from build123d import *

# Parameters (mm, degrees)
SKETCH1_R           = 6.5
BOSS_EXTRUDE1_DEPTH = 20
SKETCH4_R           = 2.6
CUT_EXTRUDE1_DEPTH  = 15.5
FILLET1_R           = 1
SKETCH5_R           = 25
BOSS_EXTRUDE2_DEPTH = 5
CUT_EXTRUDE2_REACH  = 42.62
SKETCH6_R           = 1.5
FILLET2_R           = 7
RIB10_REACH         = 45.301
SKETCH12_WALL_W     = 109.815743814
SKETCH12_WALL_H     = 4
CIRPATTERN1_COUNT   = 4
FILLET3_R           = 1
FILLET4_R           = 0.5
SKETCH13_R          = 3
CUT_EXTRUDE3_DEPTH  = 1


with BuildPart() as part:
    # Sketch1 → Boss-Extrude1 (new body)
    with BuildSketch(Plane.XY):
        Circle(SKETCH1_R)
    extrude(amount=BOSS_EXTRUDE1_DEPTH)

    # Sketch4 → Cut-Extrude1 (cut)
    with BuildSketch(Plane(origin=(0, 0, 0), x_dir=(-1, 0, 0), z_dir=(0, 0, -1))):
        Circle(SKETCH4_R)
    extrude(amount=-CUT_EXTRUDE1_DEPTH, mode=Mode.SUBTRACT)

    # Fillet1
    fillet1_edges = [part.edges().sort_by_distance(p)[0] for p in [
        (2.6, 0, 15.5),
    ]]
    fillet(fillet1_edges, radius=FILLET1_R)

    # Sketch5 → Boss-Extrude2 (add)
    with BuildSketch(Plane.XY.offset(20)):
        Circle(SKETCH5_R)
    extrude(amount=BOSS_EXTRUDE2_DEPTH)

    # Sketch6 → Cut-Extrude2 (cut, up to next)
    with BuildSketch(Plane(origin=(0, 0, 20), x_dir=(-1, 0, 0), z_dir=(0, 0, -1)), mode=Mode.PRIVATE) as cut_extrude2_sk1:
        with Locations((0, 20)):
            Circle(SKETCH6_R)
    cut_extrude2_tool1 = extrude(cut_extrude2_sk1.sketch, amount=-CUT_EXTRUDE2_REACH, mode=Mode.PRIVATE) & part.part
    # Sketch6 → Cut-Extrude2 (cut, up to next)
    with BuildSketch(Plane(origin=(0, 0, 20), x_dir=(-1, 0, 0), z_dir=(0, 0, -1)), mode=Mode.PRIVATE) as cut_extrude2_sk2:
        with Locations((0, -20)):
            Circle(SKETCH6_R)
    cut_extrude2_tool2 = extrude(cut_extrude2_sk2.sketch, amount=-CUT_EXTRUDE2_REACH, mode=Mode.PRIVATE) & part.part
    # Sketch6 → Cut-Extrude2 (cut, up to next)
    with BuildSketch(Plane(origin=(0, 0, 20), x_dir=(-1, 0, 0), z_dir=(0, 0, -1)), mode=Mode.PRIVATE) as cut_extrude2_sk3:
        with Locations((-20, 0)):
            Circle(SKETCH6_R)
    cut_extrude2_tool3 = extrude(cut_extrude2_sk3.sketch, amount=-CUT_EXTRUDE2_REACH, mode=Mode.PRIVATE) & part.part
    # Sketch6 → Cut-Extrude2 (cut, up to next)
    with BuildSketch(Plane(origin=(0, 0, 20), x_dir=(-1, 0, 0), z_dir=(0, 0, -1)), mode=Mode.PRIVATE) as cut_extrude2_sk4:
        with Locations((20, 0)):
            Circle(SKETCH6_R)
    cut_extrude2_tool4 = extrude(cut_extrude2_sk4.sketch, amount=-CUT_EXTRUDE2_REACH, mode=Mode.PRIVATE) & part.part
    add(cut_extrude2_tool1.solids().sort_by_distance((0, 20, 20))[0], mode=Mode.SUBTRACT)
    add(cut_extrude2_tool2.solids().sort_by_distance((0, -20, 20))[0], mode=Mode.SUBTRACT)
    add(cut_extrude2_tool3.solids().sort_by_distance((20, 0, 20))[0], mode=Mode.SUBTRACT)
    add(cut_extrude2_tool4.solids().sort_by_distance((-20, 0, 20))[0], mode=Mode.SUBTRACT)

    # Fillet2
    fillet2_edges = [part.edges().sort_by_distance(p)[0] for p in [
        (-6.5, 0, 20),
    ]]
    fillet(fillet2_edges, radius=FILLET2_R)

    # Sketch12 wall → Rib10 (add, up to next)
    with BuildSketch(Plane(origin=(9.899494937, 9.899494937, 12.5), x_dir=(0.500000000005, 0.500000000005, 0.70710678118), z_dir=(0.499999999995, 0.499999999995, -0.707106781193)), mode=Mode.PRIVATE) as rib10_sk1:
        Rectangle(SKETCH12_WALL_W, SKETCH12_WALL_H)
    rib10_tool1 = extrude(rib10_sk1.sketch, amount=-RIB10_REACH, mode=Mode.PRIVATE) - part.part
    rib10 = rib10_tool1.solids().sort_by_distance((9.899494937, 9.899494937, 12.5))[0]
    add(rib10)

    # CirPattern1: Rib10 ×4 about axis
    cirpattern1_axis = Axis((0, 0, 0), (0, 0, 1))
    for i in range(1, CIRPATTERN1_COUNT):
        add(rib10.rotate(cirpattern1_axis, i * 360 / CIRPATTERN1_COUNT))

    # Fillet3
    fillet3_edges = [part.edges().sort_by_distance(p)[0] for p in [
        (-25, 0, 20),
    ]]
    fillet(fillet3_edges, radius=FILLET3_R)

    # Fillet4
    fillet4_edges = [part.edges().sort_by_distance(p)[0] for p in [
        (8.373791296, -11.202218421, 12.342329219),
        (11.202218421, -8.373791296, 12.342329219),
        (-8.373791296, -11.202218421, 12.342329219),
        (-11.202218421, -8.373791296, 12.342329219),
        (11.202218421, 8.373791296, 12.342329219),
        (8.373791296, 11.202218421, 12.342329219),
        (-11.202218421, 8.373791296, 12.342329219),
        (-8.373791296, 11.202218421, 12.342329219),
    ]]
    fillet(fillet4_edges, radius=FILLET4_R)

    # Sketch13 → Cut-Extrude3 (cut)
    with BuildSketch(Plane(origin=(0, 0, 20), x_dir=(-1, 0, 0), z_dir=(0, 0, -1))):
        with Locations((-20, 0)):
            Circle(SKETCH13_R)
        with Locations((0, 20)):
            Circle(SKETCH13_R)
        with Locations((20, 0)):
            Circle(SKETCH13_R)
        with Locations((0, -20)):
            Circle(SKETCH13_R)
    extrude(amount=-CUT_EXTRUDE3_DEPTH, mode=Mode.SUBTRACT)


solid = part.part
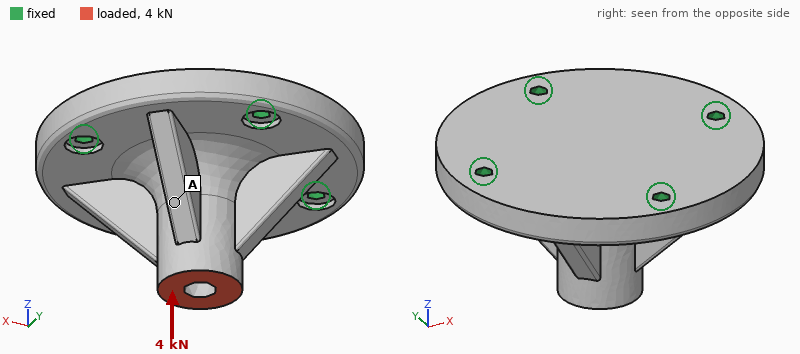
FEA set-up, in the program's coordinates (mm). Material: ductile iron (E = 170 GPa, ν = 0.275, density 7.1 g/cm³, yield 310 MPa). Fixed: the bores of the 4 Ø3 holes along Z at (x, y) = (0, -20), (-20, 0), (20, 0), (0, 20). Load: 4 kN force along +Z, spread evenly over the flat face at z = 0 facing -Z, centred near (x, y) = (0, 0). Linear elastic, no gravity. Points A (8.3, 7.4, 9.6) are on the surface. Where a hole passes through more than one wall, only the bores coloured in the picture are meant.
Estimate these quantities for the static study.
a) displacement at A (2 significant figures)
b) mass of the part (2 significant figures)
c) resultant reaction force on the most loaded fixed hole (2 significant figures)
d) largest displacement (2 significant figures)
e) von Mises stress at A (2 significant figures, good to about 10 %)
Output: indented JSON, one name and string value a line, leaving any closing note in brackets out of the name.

{
  "displacement at A": "7.1 µm",
  "mass of the part": "100 g",
  "resultant reaction force on the most loaded fixed hole": "1.1 kN",
  "largest displacement": "9.9 µm",
  "von Mises stress at A": "25 MPa"
}
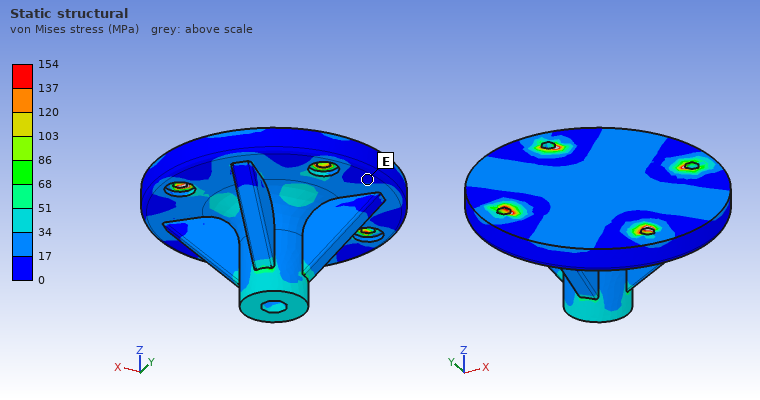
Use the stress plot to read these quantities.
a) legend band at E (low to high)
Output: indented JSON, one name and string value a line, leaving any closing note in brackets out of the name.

{
  "legend band at E": "0 to 17 MPa"
}
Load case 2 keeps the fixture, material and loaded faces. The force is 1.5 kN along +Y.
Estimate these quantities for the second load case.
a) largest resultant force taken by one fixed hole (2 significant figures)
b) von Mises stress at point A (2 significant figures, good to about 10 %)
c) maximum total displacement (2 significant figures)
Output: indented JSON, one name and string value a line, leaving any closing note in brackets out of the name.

{
  "largest resultant force taken by one fixed hole": "1.0 kN",
  "von Mises stress at point A": "30 MPa",
  "maximum total displacement": "17 µm"
}
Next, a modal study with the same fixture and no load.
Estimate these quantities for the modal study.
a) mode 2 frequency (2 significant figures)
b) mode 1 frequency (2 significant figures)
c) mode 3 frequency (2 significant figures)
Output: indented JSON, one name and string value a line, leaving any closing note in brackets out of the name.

{
  "mode 2 frequency": "15 kHz",
  "mode 1 frequency": "15 kHz",
  "mode 3 frequency": "15 kHz"
}
